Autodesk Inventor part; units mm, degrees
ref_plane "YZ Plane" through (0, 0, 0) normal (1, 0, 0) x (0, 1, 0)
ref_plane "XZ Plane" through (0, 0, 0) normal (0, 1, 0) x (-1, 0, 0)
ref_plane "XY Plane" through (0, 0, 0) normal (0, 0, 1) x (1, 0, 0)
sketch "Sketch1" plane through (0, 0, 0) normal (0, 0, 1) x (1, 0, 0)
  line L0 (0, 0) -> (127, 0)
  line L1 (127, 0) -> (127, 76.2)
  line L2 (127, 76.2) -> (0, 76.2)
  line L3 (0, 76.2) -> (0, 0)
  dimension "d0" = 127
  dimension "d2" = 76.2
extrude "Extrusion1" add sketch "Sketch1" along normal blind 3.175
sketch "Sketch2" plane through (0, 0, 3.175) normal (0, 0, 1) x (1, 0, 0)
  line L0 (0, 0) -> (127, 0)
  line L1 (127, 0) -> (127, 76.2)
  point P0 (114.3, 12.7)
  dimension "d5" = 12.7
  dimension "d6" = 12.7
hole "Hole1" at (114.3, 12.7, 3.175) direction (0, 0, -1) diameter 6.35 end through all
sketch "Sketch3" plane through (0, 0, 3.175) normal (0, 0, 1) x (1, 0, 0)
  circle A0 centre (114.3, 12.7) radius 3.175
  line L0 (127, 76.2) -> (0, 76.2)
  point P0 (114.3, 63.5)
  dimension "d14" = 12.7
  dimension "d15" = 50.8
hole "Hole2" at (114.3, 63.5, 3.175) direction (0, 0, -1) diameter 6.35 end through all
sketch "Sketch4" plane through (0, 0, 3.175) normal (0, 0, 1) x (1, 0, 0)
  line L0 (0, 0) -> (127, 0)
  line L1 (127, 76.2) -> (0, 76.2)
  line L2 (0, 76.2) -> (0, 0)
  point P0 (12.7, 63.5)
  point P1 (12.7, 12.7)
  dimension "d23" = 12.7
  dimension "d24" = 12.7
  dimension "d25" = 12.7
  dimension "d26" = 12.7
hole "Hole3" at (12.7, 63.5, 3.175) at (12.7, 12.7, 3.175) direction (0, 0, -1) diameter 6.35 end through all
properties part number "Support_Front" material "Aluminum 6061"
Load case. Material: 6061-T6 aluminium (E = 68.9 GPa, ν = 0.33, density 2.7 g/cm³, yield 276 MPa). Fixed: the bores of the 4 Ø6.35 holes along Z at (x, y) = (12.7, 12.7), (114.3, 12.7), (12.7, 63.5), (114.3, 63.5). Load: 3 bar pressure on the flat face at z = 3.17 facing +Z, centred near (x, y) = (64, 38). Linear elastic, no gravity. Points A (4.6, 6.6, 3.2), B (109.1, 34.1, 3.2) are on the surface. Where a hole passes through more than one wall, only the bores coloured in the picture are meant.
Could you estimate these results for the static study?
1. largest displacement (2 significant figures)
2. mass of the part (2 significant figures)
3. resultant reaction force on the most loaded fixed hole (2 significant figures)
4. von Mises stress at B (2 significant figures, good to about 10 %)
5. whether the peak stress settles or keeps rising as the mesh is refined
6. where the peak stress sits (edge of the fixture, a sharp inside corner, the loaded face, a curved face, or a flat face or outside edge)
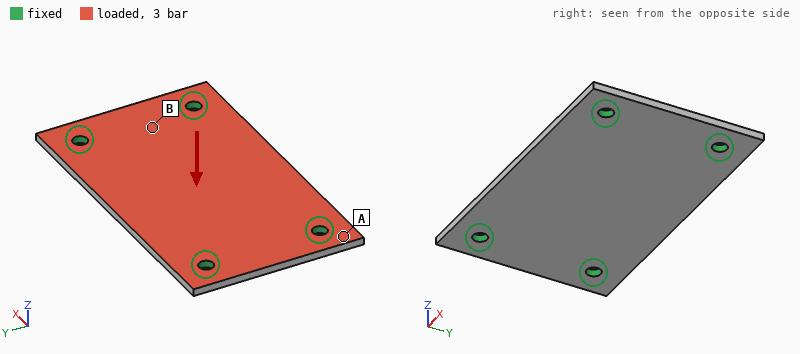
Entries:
0.47 mm
82 g
720 N
51 MPa
keeps rising
edge of the fixture
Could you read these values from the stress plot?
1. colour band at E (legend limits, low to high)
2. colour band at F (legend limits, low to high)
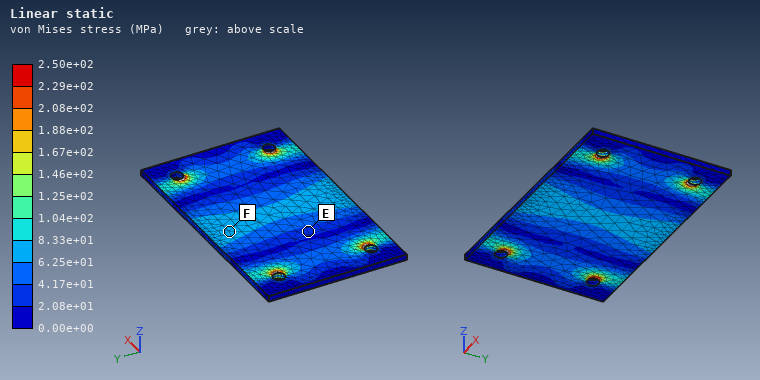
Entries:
2.08e+01 to 4.17e+01 MPa
6.25e+01 to 8.33e+01 MPa
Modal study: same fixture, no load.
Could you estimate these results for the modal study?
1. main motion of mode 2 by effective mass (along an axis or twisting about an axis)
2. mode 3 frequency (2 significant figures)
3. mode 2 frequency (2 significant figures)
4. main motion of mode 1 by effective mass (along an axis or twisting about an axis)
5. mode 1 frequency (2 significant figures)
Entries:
twisting about X
4100 Hz
2200 Hz
along Z
1600 Hz
